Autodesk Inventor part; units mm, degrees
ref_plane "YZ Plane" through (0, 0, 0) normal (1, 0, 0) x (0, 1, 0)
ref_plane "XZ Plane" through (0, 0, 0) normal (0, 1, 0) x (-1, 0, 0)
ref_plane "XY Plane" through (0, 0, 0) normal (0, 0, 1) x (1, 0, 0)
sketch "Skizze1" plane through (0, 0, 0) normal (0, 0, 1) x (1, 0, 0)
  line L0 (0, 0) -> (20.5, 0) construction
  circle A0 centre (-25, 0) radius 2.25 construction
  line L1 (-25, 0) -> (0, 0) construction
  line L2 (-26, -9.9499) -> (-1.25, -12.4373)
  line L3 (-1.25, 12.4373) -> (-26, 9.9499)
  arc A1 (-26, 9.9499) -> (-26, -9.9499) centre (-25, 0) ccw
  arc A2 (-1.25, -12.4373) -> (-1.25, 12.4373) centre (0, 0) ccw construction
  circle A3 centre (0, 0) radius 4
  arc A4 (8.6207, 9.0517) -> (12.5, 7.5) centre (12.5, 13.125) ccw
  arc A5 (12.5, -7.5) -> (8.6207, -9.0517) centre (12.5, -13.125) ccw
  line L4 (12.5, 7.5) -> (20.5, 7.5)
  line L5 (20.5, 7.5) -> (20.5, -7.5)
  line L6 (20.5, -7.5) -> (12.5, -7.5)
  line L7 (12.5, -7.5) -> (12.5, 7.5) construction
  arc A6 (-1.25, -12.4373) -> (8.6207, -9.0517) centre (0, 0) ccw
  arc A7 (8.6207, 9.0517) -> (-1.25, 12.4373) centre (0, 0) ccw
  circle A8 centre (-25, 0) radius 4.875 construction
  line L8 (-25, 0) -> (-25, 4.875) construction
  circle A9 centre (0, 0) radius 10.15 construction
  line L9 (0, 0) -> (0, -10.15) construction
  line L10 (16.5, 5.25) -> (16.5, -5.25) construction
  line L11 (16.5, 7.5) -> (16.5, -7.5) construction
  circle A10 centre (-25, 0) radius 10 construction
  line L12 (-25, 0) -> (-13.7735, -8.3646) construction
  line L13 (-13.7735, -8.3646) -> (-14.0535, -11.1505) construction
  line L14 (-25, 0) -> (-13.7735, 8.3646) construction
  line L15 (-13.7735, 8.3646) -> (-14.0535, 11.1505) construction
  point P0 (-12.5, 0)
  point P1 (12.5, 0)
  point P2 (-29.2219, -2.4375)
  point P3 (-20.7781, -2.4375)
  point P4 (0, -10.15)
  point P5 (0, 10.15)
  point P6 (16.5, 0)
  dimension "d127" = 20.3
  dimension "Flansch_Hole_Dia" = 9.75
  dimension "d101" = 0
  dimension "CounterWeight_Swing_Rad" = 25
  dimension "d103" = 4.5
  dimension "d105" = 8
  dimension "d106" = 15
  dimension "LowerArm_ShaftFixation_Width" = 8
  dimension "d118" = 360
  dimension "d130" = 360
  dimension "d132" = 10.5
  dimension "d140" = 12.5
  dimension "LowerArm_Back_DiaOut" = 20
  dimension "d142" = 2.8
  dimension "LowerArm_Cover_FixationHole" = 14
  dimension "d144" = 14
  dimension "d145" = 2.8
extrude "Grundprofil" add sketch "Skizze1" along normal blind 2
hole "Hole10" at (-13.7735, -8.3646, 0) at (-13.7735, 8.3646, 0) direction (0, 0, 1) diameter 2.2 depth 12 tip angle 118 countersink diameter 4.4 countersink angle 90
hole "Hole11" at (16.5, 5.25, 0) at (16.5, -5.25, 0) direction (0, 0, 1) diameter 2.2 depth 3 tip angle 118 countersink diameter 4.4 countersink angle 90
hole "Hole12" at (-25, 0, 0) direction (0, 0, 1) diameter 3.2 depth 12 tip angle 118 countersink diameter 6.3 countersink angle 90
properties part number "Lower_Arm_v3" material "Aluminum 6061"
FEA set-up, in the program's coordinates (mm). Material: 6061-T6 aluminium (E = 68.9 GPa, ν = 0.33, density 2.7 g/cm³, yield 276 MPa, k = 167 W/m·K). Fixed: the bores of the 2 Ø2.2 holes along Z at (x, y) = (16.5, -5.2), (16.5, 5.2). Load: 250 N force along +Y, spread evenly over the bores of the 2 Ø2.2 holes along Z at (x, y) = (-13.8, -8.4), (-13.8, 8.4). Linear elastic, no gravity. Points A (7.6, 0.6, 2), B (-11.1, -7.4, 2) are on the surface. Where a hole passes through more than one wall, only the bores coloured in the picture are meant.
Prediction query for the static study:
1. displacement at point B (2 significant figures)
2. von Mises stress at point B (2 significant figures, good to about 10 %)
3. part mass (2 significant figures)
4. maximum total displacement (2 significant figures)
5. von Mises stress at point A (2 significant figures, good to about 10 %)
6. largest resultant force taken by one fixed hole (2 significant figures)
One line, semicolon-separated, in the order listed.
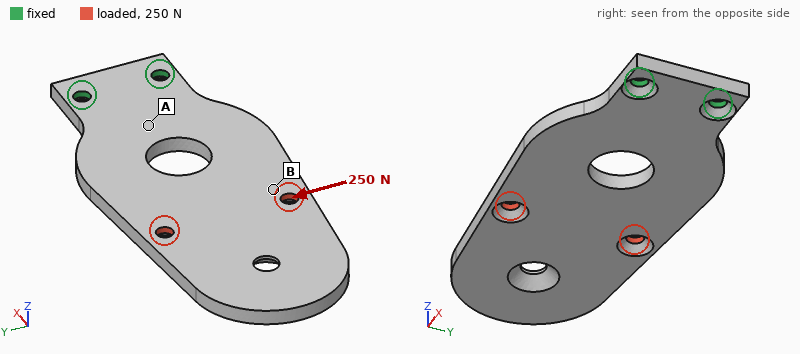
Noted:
0.080 mm; 21 MPa; 5.4 g; 0.13 mm; 64 MPa; 680 N
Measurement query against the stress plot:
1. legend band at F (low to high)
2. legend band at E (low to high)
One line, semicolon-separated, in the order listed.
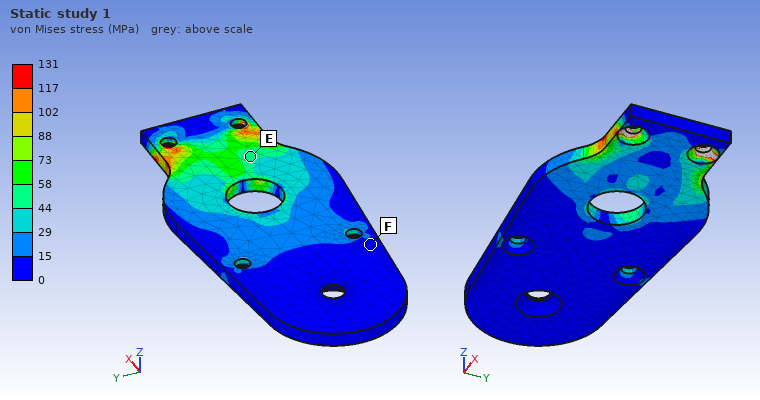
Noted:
0 to 15 MPa; 44 to 58 MPa
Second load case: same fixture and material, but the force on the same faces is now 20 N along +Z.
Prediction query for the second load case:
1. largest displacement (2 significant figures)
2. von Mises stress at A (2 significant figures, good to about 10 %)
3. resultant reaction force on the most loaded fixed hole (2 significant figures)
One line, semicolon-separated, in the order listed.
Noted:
0.60 mm; 29 MPa; 23 N
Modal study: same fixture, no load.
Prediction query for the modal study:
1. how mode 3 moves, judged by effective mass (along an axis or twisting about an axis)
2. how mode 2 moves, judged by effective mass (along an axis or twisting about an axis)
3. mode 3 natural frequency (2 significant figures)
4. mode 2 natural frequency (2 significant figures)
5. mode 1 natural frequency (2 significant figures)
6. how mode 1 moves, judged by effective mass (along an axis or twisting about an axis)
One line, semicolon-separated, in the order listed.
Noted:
along Z; twisting about X; 3600 Hz; 2800 Hz; 560 Hz; along Z
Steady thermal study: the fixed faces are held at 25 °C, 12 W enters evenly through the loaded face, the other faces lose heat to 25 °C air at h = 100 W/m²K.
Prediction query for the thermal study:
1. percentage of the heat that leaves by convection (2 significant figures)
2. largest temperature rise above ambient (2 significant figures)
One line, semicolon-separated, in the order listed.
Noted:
49 %; 43 K
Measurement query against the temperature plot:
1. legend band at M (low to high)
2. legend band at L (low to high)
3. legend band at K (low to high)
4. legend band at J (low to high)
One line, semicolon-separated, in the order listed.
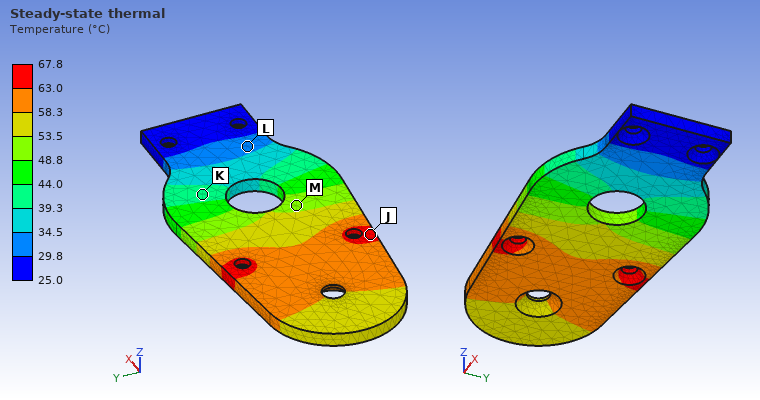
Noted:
48.8 to 53.5 °C; 29.8 to 34.5 °C; 39.3 to 44.0 °C; 63.0 to 67.8 °C
